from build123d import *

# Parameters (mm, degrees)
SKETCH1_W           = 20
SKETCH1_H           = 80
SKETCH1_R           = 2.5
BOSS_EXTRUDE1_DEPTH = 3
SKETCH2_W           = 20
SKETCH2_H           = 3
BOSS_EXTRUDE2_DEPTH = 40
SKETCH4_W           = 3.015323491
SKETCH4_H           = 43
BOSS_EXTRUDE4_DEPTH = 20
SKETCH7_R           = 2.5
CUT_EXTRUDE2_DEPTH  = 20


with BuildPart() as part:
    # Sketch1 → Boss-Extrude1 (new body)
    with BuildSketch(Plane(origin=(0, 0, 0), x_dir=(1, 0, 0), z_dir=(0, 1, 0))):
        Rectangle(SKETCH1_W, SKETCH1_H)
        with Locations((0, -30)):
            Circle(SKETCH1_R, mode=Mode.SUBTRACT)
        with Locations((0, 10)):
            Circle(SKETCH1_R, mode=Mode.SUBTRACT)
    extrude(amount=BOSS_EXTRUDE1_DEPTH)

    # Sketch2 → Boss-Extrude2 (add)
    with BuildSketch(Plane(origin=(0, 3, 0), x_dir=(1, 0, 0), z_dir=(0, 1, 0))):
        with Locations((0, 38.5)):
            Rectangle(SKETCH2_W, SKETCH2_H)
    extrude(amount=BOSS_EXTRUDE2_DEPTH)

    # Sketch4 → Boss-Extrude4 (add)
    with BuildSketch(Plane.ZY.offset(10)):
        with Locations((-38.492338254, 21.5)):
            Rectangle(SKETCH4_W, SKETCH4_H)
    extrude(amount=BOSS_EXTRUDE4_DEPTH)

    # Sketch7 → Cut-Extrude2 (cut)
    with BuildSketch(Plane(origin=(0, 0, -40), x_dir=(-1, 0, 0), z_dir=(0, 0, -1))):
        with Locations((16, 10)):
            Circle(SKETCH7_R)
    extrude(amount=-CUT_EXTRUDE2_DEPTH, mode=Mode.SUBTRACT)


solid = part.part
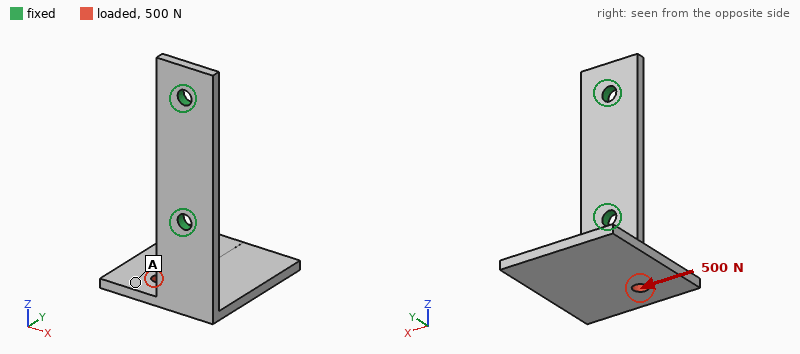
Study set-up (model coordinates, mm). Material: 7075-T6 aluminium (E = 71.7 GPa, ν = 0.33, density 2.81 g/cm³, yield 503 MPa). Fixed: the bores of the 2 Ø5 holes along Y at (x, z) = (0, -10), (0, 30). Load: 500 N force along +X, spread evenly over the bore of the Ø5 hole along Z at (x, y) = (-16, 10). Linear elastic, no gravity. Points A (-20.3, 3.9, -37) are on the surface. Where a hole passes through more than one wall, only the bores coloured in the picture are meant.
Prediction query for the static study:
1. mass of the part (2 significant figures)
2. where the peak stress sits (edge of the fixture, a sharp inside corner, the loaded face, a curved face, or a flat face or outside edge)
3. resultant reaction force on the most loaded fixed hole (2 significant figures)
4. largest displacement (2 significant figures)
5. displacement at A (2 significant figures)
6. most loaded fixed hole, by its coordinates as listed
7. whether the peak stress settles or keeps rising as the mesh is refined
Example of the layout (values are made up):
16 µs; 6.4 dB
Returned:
27 g; edge of the fixture; 720 N; 1.2 mm; 0.46 mm; (0, -10); keeps rising
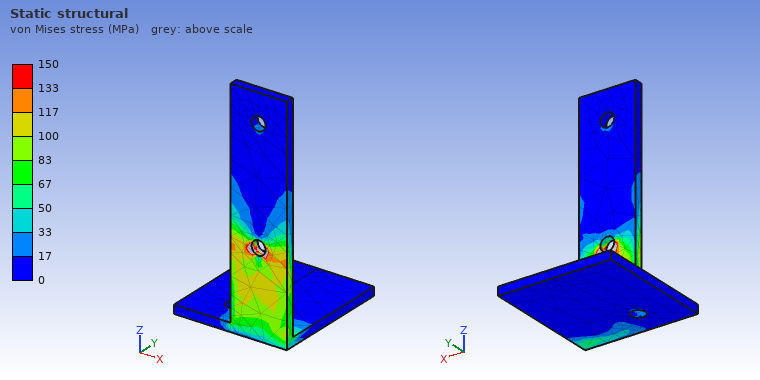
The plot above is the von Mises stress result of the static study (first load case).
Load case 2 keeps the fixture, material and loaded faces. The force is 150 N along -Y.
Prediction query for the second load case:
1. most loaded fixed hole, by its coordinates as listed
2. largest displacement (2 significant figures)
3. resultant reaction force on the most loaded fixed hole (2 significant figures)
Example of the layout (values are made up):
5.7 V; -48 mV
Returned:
(0, -10); 1.2 mm; 150 N
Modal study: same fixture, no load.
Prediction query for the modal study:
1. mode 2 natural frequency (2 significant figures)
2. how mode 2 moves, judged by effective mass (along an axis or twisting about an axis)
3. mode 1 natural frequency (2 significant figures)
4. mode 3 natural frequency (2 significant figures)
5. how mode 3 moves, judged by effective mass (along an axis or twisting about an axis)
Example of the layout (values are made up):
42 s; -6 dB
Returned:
670 Hz; along X; 480 Hz; 1600 Hz; along Y
